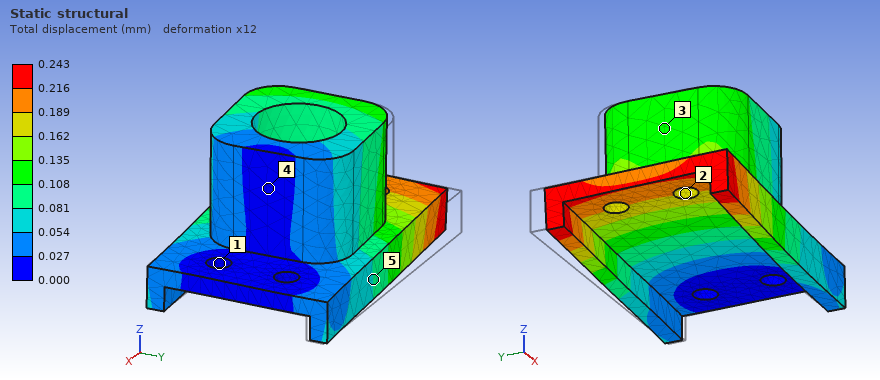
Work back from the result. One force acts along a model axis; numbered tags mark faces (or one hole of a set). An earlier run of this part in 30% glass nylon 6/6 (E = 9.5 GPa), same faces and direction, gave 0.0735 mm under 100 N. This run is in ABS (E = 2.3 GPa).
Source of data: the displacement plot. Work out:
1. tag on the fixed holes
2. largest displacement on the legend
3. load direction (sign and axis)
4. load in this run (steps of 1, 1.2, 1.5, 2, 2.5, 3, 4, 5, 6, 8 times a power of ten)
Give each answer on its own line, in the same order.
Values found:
1
0.243 mm
-Y
80 N
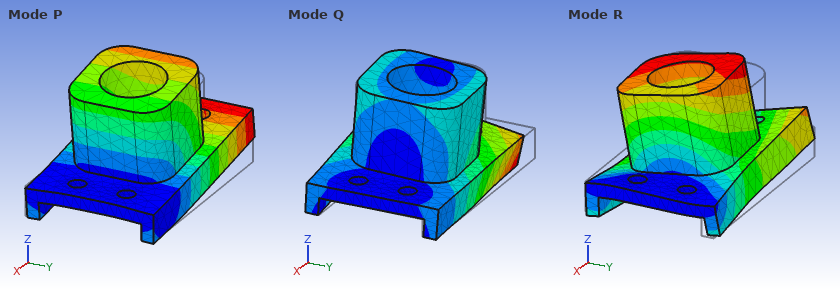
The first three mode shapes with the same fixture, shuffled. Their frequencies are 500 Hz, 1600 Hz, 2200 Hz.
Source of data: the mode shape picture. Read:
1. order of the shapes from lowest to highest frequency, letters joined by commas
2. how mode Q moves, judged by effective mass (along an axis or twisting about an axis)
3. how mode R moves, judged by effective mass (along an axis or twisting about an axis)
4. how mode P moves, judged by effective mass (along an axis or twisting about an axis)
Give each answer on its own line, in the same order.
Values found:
P, R, Q
along Y
along Y
along Z
